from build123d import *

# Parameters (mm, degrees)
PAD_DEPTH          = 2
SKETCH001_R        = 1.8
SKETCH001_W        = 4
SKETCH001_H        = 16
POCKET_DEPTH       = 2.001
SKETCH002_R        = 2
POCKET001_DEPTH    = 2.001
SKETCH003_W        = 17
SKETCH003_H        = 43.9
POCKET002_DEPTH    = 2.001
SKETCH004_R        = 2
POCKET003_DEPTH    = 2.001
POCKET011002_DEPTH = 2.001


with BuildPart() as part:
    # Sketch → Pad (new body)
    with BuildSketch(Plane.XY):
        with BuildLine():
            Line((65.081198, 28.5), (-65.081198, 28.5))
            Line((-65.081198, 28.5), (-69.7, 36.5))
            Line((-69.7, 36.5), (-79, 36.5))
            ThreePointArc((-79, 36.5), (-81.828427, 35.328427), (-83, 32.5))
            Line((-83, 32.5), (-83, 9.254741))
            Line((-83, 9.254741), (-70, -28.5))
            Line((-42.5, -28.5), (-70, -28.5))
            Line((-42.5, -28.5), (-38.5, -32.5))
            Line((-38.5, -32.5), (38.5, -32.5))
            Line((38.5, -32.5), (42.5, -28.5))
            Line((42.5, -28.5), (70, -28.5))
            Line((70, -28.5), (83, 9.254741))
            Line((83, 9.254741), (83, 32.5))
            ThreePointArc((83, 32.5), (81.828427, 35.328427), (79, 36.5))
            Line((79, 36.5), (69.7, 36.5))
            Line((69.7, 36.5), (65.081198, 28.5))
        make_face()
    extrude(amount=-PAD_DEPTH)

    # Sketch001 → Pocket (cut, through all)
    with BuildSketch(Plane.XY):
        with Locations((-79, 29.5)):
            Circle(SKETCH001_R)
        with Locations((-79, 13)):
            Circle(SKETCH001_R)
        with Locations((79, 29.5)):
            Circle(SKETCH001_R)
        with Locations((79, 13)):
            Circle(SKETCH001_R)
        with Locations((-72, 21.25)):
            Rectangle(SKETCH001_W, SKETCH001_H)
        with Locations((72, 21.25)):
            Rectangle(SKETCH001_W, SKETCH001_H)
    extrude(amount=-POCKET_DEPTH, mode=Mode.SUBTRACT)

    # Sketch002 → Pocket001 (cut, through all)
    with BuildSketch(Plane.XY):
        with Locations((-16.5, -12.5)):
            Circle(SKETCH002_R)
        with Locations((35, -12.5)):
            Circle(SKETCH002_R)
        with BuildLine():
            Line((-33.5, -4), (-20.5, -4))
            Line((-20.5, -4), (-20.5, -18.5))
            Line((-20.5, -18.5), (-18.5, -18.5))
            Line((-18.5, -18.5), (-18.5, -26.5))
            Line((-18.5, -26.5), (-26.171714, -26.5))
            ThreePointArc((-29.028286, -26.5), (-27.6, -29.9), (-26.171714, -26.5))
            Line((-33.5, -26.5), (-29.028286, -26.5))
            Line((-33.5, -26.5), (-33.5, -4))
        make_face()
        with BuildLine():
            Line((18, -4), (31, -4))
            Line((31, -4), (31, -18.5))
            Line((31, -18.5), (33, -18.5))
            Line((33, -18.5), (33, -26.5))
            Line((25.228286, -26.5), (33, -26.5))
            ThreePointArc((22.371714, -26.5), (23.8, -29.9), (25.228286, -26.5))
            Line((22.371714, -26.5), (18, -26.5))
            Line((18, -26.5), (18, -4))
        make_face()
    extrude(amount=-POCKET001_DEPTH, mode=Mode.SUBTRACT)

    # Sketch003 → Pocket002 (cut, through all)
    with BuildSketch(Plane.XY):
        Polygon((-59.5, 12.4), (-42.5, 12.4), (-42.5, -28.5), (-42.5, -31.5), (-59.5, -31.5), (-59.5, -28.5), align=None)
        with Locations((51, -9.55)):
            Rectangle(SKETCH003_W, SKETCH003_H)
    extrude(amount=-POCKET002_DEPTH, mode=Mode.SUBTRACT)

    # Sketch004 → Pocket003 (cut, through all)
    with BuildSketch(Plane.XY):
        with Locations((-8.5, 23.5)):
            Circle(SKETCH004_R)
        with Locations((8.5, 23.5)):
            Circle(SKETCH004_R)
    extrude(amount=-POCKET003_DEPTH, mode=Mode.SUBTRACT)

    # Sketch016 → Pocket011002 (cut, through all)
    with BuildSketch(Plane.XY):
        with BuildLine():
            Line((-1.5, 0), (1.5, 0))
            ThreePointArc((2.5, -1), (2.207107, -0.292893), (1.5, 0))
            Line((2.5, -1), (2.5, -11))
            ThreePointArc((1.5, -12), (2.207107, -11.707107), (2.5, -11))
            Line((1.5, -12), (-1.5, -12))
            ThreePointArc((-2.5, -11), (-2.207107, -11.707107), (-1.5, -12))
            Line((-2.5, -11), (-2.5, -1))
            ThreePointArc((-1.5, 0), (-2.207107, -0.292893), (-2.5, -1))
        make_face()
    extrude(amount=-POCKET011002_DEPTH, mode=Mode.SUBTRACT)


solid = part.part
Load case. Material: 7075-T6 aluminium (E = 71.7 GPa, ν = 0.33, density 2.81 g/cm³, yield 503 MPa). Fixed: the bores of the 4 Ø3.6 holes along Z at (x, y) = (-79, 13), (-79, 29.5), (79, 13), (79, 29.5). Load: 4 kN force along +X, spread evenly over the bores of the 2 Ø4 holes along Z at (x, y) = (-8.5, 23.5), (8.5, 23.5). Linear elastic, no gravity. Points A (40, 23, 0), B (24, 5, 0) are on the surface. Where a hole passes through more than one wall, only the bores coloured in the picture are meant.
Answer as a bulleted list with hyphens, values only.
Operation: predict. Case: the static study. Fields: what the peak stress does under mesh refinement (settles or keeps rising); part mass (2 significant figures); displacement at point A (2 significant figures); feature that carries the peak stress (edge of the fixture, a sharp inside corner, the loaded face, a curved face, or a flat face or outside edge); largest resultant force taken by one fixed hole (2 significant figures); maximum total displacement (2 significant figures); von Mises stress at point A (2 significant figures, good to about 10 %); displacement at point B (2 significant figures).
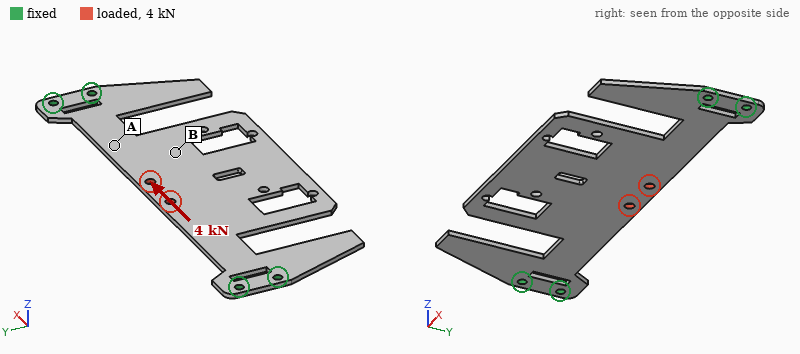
- keeps rising
- 41 g
- 53 µm
- edge of the fixture
- 1.4 kN
- 88 µm
- 64 MPa
- 61 µm
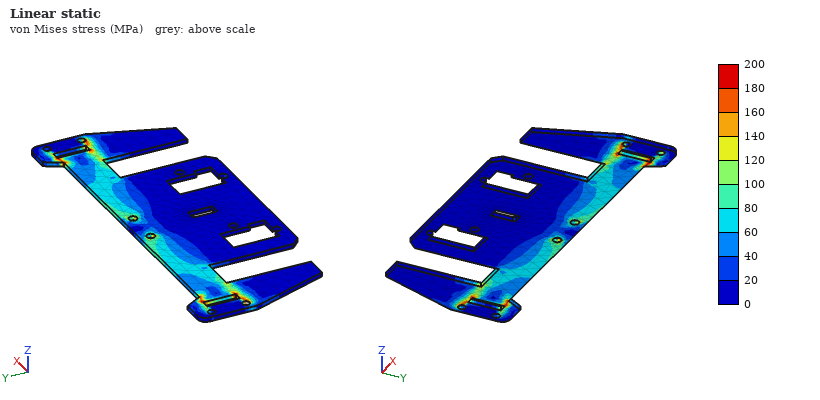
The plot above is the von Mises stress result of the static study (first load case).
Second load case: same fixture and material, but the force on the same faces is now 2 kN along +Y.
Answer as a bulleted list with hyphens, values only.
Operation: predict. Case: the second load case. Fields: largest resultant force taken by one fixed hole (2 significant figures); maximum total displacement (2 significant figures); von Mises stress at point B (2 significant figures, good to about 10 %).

- 1.5 kN
- 0.24 mm
- 56 MPa
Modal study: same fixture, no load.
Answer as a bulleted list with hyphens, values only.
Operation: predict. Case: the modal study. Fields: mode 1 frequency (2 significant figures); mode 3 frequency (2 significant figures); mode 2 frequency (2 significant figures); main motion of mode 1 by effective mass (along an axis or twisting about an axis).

- 220 Hz
- 720 Hz
- 530 Hz
- along Z
